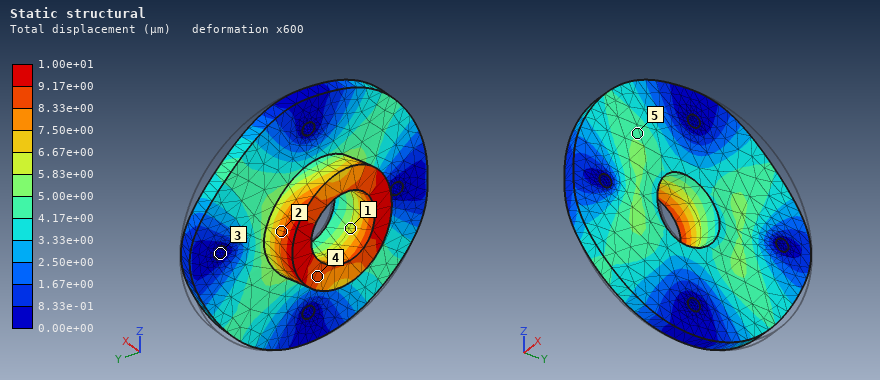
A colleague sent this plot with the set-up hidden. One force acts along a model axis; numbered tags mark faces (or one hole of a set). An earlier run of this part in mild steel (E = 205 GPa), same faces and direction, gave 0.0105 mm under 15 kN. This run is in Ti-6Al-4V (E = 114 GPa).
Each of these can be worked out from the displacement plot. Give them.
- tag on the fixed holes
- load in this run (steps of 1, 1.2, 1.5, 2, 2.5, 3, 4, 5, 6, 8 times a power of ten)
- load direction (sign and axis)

3
8 kN
-Y
